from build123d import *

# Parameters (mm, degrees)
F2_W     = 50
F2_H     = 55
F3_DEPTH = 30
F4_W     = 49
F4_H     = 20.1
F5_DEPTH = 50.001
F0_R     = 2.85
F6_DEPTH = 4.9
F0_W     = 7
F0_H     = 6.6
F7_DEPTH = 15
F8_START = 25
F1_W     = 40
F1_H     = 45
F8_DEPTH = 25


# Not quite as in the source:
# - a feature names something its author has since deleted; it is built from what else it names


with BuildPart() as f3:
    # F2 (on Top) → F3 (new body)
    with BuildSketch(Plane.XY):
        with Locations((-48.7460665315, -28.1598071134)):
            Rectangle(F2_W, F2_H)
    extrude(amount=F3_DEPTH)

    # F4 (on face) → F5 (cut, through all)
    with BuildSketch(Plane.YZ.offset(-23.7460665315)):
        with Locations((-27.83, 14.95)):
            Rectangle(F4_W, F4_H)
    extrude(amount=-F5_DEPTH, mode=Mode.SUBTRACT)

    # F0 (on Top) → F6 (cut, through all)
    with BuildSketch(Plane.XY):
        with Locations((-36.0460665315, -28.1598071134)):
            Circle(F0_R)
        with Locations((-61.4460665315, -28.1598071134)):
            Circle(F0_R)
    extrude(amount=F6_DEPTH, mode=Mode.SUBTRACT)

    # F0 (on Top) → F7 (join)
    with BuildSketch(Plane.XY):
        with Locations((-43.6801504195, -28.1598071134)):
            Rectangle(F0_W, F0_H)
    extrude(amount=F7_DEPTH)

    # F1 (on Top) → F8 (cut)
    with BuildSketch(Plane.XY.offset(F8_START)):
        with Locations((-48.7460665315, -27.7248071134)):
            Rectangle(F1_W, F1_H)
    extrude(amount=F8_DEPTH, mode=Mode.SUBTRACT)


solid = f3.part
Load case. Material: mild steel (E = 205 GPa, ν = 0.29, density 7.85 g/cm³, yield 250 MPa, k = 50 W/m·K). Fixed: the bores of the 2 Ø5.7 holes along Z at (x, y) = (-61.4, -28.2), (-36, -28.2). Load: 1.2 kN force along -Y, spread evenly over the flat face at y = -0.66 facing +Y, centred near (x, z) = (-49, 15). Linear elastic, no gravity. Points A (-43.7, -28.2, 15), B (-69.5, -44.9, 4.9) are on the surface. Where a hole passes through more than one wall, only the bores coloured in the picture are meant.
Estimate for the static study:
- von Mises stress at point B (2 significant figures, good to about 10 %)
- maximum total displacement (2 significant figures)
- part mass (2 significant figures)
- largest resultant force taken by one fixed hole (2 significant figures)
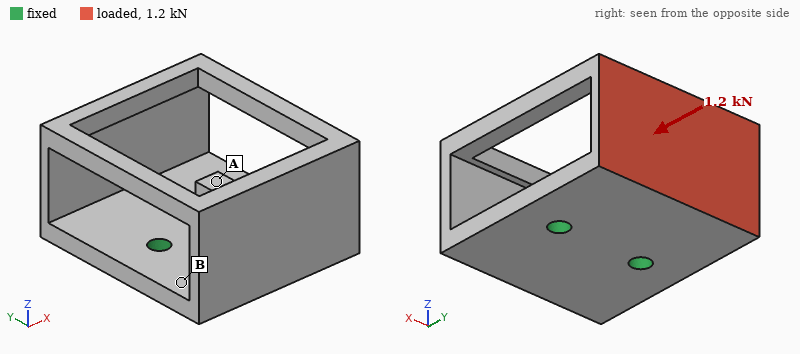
28 MPa
81 µm
190 g
610 N
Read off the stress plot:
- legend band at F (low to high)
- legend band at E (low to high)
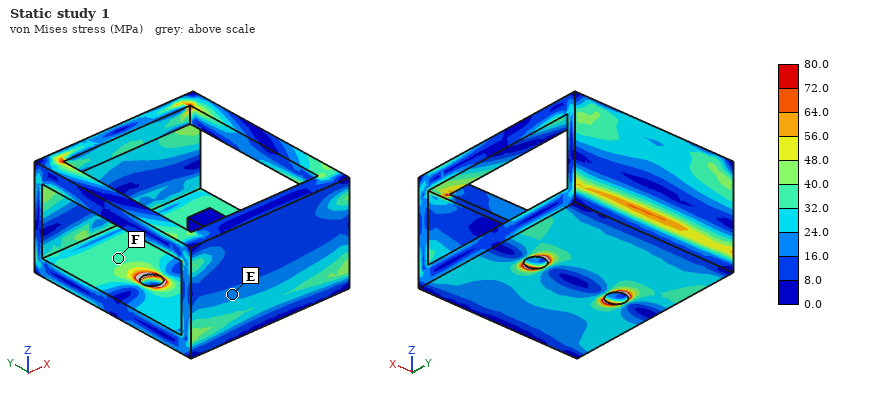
32.0 to 40.0 MPa
16.0 to 24.0 MPa
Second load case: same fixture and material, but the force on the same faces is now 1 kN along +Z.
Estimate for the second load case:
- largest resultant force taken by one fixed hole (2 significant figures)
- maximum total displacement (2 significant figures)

510 N
71 µm
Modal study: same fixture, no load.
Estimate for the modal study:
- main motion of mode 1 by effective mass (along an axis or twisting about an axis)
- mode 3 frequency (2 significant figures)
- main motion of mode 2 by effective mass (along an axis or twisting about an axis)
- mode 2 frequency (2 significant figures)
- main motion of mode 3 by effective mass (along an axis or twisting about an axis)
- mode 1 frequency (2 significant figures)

along Y
3400 Hz
along X
3000 Hz
along Z
1900 Hz
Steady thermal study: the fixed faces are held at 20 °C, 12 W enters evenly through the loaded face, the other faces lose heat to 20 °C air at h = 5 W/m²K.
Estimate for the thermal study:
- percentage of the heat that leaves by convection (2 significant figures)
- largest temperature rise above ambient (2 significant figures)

6.5 %
38 K
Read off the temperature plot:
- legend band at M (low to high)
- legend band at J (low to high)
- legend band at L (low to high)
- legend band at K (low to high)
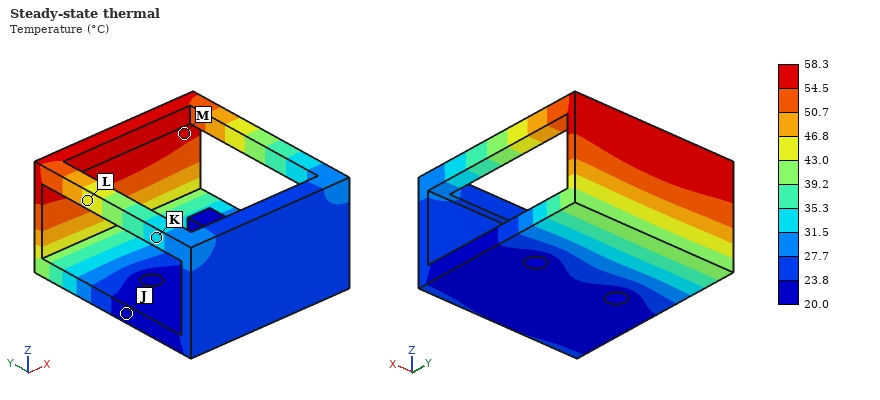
54.5 to 58.3 °C
20.0 to 23.8 °C
43.0 to 46.8 °C
31.5 to 35.3 °C
